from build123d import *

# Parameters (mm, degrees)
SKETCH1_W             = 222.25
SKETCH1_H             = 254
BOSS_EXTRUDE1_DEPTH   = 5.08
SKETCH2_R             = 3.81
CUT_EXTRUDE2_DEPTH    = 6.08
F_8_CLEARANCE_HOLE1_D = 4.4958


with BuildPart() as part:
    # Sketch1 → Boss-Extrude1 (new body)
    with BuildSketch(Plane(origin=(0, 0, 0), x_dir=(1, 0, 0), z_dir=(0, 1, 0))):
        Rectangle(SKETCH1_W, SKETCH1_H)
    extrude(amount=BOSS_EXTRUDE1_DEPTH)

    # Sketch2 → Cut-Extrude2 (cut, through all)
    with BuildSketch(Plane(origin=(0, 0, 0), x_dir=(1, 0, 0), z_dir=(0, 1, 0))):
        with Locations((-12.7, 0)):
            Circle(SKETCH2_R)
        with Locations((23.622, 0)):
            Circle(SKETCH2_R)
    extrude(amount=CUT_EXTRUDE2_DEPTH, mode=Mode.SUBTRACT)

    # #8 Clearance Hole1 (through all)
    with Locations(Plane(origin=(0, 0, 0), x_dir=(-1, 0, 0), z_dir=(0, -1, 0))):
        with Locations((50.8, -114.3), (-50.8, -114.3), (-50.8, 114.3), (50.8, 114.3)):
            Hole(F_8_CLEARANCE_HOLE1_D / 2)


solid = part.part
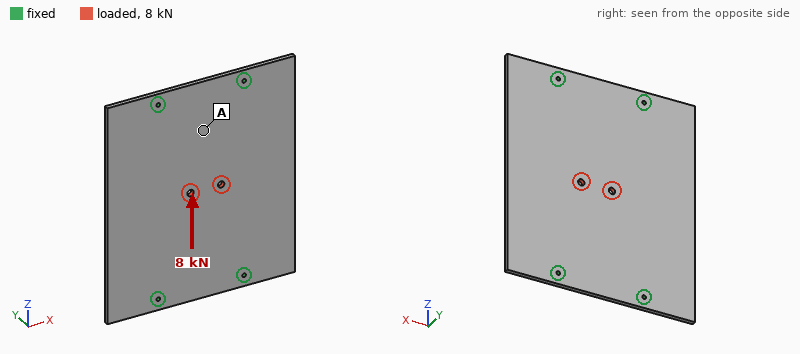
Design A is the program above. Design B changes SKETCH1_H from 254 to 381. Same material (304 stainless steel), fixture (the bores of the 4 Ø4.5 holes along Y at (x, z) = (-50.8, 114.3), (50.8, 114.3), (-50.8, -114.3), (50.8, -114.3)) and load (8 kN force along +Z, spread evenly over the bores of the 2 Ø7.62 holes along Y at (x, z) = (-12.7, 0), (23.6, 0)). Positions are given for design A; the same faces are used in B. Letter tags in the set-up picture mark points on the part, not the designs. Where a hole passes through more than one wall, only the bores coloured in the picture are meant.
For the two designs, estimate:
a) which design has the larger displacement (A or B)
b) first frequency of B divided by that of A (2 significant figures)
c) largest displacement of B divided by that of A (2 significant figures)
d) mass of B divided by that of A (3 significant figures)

A
0.96
0.92
1.50
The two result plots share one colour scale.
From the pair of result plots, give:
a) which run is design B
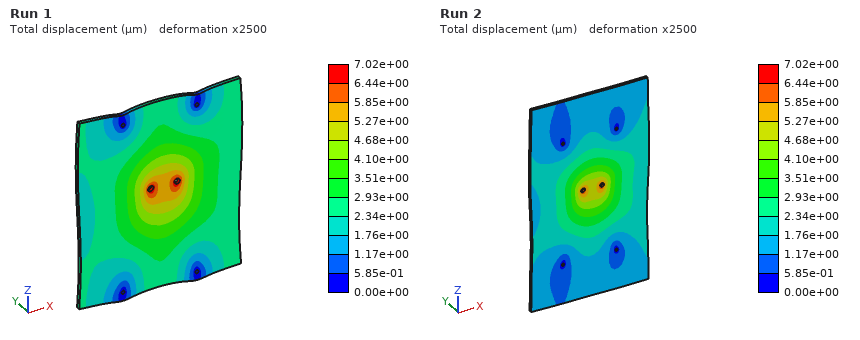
Run 2
